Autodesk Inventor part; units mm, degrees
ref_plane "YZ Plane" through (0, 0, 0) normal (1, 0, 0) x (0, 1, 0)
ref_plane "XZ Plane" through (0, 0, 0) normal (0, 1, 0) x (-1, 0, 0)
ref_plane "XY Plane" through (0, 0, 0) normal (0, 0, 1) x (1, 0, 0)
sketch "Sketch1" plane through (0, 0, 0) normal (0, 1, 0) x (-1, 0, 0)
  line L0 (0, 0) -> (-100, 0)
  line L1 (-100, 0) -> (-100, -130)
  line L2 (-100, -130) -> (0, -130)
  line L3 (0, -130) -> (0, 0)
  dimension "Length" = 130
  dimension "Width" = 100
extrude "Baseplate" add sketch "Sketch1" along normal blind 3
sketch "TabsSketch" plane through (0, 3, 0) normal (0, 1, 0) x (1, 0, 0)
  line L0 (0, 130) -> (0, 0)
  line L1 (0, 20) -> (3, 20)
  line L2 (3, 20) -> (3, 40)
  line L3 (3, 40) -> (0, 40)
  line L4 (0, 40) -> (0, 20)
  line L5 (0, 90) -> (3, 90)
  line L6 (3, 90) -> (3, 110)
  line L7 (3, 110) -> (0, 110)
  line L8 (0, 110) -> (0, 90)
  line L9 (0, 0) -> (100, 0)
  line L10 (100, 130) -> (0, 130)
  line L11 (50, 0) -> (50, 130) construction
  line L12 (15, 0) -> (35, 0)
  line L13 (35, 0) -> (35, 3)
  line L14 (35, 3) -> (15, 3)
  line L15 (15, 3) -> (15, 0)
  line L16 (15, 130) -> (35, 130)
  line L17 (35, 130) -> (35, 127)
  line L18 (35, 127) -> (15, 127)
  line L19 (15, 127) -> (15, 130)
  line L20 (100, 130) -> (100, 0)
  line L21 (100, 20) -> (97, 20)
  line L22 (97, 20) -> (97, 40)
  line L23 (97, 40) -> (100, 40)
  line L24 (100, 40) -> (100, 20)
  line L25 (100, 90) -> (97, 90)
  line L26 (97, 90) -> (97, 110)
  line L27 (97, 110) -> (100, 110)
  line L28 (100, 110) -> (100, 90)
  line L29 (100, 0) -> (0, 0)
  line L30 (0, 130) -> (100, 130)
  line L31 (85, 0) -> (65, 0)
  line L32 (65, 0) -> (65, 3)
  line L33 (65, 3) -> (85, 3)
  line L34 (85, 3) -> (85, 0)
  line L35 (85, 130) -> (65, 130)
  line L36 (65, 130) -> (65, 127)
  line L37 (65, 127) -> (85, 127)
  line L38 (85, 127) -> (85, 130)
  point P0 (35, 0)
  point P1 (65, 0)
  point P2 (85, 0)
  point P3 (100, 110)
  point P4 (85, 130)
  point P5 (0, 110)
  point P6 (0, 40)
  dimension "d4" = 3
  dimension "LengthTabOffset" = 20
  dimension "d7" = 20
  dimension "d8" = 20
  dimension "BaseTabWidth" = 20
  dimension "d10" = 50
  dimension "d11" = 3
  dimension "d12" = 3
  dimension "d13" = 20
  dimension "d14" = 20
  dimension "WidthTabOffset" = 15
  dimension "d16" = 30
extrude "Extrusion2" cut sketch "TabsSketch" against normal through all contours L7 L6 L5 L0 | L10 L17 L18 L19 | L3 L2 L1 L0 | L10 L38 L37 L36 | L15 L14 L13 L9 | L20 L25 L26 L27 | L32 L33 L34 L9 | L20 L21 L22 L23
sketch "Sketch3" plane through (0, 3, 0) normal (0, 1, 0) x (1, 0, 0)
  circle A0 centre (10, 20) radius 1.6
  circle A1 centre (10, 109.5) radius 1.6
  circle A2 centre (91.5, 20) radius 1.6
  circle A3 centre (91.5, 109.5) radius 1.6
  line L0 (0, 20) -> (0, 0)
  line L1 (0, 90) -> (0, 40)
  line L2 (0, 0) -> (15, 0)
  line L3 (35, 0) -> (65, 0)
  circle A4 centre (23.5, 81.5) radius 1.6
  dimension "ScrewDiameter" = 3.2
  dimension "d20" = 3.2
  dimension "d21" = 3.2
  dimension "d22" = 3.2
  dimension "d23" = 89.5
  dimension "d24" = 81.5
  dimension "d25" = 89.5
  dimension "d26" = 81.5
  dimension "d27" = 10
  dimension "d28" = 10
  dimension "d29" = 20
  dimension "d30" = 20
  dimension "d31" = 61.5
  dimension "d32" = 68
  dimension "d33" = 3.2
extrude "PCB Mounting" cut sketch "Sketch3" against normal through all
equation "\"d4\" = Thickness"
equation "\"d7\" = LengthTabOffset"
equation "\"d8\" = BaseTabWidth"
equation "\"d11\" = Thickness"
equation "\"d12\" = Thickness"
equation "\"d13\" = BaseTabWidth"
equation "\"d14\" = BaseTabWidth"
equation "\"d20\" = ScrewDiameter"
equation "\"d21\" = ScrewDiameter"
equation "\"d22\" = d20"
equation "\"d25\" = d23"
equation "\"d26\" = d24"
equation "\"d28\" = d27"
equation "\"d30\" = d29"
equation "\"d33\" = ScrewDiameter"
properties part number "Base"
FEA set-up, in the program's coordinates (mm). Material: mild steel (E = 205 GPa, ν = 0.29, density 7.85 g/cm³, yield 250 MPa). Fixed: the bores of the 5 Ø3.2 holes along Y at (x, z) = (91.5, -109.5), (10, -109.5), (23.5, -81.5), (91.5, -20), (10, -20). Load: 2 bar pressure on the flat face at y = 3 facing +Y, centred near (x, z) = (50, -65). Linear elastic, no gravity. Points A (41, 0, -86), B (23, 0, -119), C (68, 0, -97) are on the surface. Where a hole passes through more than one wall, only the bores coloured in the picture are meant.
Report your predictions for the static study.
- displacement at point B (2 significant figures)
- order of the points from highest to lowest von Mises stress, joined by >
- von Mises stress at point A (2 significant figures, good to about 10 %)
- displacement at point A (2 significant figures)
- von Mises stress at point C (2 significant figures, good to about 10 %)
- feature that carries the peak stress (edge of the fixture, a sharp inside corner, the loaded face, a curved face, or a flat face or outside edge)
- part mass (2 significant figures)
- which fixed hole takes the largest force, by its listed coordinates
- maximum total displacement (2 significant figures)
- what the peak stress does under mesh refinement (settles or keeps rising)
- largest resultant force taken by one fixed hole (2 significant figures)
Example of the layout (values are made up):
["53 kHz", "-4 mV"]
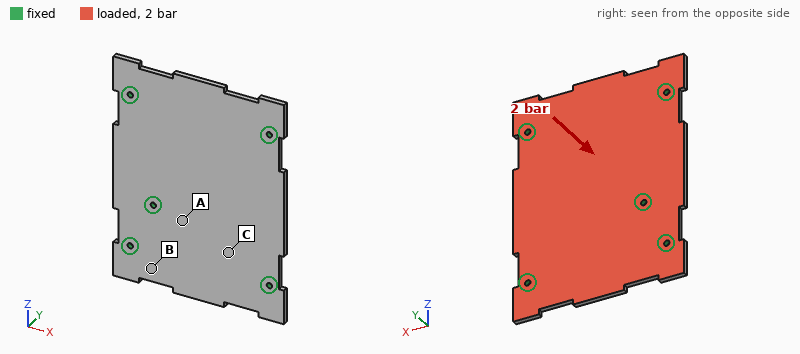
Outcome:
["21 µm", "C > A > B", "33 MPa", "35 µm", "43 MPa", "edge of the fixture", "290 g", "(23.5, -81.5)", "94 µm", "keeps rising", "710 N"]
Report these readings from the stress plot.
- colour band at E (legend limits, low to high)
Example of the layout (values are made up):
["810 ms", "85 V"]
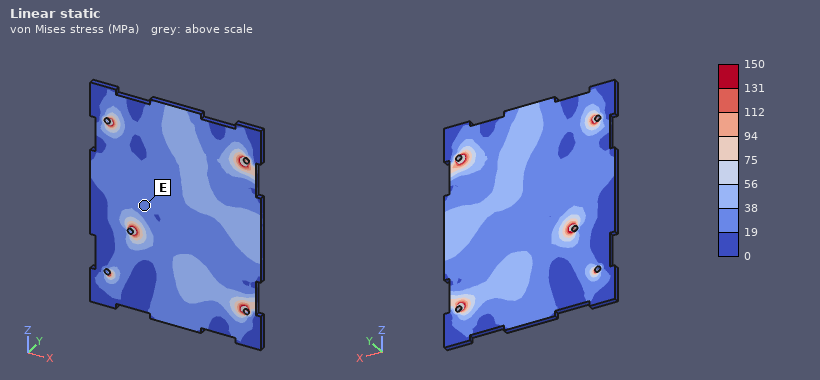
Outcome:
["19 to 38 MPa"]
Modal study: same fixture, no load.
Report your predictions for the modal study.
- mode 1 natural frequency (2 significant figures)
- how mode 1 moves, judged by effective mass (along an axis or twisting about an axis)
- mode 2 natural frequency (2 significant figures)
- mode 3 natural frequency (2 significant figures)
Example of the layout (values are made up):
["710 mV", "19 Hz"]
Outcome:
["1700 Hz", "along Y", "2100 Hz", "2200 Hz"]
